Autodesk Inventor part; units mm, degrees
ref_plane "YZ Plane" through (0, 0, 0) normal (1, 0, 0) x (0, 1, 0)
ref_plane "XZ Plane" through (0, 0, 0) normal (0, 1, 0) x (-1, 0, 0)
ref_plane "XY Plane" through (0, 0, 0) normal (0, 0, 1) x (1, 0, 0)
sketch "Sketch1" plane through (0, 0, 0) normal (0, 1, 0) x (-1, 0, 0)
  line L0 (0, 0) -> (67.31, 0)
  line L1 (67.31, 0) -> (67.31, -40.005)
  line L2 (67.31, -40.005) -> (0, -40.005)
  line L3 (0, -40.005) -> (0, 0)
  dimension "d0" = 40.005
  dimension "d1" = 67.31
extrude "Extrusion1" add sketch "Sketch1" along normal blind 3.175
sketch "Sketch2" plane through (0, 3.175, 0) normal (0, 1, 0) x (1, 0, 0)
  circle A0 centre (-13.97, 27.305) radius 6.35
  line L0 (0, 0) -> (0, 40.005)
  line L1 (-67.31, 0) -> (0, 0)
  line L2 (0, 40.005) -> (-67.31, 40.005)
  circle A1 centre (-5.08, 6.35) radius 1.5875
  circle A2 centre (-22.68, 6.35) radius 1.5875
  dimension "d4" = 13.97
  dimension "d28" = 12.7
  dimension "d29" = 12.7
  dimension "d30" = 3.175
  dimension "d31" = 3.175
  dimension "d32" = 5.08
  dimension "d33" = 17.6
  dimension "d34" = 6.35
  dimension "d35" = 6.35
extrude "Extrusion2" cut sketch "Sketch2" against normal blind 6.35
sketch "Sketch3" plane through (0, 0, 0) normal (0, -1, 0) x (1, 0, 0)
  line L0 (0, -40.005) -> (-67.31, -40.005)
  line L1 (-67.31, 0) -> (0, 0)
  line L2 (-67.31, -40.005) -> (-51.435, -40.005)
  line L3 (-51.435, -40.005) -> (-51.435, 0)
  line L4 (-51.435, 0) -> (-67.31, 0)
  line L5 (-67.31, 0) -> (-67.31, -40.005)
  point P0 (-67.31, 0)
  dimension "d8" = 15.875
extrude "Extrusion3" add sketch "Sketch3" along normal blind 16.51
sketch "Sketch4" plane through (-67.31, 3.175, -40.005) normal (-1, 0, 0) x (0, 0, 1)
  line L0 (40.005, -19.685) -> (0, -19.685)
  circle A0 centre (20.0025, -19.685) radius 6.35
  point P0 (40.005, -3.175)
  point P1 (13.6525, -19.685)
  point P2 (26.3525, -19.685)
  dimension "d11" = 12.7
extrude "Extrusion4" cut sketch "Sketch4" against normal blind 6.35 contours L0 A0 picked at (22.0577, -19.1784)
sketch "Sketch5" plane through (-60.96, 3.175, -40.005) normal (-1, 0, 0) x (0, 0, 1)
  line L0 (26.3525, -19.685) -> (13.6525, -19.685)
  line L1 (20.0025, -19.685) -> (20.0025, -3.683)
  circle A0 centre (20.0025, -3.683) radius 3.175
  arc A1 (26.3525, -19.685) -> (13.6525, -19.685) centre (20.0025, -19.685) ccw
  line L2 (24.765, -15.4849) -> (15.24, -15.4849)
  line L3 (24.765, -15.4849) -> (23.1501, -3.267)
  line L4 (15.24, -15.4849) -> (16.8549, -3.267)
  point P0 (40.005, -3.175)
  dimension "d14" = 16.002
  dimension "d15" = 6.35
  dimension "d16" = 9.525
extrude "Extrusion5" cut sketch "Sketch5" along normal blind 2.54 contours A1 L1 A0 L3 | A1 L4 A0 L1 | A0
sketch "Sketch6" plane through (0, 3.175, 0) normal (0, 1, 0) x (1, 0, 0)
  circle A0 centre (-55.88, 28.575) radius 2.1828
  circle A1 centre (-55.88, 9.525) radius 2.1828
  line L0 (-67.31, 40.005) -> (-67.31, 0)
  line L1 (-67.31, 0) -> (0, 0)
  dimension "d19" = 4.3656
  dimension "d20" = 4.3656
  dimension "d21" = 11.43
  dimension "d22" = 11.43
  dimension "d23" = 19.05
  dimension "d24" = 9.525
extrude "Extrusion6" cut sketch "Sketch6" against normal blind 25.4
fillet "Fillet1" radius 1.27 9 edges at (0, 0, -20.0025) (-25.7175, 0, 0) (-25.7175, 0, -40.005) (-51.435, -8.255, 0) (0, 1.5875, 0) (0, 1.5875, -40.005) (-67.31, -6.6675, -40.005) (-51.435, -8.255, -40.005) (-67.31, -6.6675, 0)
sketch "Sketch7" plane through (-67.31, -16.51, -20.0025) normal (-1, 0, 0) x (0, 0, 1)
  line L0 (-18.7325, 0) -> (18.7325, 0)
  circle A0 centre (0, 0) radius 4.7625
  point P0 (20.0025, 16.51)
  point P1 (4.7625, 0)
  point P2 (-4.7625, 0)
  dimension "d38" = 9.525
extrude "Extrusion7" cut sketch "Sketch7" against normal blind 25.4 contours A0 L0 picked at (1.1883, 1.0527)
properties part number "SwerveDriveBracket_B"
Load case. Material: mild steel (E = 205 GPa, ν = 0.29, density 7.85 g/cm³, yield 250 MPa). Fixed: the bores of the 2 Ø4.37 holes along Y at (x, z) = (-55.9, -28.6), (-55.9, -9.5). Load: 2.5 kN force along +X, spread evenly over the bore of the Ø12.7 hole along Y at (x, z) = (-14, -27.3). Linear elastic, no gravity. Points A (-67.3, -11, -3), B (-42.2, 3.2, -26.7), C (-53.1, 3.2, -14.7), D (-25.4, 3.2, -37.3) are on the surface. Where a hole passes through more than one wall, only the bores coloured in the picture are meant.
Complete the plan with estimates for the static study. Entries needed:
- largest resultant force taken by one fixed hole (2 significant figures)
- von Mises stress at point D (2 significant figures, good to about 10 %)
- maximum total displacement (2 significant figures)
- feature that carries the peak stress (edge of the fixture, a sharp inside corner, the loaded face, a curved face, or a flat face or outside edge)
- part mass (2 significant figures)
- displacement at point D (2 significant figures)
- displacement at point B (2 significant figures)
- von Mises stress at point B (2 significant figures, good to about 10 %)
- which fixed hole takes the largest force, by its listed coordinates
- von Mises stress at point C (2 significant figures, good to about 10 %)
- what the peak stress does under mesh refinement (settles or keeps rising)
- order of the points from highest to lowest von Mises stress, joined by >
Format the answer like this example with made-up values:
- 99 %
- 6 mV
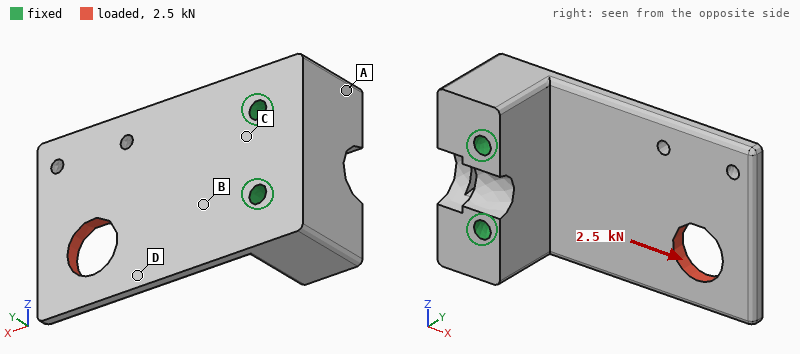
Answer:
- 2.1 kN
- 40 MPa
- 14 µm
- edge of the fixture
- 130 g
- 8.4 µm
- 2.7 µm
- 29 MPa
- (-55.9, -28.6)
- 13 MPa
- keeps rising
- D > B > C > A
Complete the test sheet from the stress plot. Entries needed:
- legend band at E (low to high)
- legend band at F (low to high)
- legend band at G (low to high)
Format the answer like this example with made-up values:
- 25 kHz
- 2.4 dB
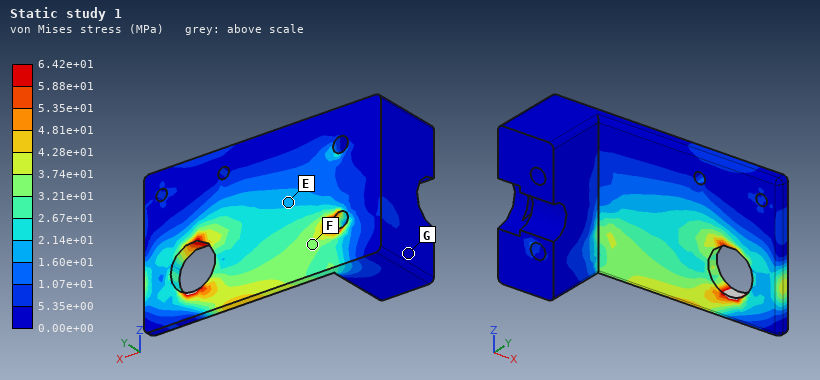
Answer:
- 1.60e+01 to 2.14e+01 MPa
- 3.21e+01 to 3.74e+01 MPa
- 0.00e+00 to 5.35e+00 MPa
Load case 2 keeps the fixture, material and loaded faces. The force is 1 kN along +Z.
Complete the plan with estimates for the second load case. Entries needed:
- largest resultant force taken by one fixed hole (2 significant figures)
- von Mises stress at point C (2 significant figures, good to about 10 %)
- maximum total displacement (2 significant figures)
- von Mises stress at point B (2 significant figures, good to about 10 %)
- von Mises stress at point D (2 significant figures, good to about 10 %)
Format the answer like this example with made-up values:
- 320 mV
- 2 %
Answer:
- 1.8 kN
- 13 MPa
- 20 µm
- 21 MPa
- 14 MPa
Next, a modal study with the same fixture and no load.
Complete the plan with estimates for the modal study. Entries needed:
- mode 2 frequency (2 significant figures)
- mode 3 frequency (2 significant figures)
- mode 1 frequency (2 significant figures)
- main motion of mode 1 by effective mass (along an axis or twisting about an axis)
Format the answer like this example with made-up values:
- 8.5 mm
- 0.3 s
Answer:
- 2800 Hz
- 5500 Hz
- 1000 Hz
- along Y
